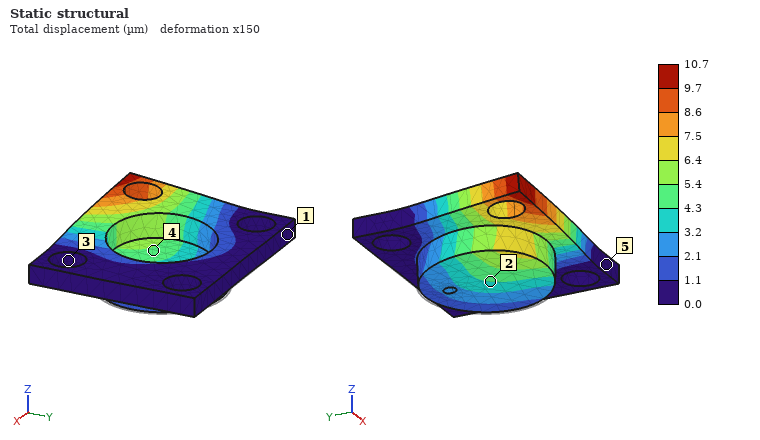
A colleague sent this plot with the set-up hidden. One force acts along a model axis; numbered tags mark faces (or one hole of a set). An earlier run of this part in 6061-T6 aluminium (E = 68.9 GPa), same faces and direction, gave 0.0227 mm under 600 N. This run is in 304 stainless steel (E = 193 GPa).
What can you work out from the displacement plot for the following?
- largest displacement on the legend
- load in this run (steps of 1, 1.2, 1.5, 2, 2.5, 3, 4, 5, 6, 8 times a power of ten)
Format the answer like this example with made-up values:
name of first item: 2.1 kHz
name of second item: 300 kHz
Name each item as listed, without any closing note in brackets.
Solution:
largest displacement on the legend: 10.7 µm
load in this run: 800 N
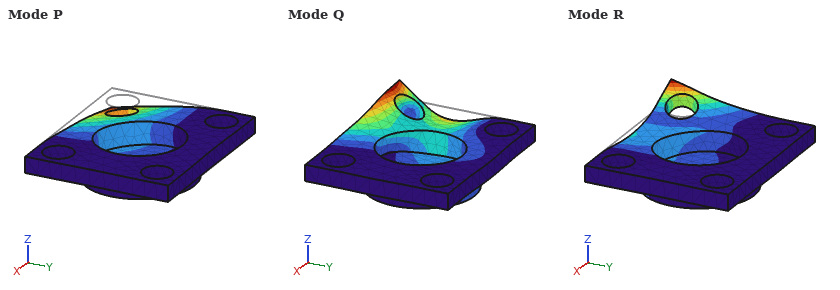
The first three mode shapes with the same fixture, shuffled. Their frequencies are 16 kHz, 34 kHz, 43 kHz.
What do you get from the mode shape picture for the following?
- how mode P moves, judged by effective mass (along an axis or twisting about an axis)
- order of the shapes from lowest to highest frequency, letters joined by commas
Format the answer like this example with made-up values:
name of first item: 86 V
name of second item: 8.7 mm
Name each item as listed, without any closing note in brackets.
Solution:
how mode P moves, judged by effective mass: along Z
order of the shapes from lowest to highest frequency, letters joined by commas: P, R, Q
